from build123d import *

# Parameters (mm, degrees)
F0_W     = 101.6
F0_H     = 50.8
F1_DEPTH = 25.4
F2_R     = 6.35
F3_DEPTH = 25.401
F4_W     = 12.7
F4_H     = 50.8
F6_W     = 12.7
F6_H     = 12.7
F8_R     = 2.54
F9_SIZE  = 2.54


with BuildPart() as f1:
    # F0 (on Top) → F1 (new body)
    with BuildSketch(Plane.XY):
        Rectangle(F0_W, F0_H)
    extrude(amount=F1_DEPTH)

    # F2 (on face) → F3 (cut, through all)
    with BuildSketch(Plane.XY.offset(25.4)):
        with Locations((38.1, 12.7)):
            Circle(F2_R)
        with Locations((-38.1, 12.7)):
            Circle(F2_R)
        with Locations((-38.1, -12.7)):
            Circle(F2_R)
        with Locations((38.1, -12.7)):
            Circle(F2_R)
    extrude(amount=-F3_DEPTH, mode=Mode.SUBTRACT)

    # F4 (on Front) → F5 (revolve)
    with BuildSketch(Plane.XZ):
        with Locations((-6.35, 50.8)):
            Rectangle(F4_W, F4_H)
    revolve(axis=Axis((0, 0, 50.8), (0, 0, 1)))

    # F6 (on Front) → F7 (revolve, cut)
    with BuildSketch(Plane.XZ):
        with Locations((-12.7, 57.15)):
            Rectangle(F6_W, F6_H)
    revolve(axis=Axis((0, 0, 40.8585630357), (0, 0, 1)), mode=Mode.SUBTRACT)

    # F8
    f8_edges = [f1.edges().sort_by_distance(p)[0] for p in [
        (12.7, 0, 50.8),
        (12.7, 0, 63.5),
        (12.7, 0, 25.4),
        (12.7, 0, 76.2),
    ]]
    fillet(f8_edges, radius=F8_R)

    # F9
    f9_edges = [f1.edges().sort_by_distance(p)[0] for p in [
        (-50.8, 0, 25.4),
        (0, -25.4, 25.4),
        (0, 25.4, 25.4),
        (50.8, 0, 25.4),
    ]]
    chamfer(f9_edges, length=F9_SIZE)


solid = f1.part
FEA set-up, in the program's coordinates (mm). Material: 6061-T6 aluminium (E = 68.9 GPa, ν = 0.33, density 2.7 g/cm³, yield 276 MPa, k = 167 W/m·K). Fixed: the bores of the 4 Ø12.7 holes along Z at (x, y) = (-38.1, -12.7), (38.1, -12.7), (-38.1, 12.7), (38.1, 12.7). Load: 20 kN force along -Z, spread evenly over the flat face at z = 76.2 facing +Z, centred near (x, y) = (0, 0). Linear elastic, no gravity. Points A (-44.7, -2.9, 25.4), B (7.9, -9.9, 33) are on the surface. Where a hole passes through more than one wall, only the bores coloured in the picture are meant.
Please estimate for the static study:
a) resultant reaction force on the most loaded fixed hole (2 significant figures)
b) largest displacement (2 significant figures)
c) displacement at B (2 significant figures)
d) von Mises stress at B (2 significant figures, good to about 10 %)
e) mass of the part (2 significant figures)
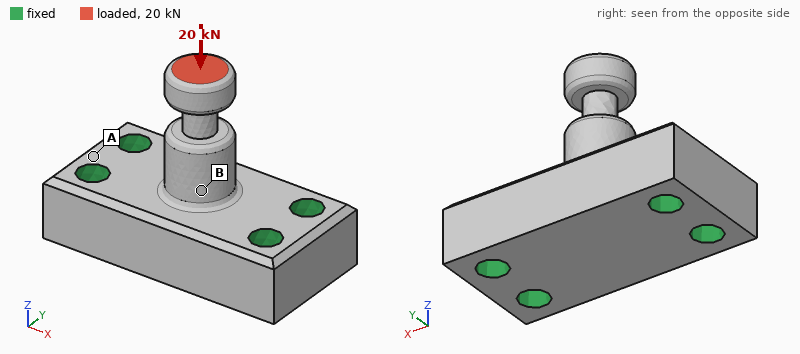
5.1 kN
81 µm
20 µm
37 MPa
370 g
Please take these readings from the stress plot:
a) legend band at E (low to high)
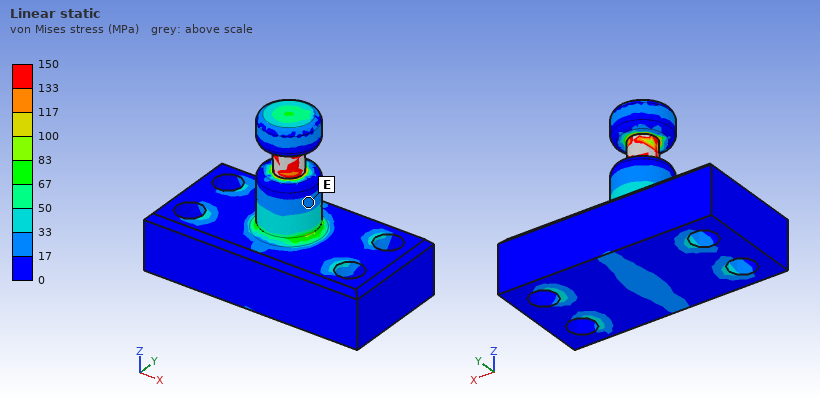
17 to 33 MPa
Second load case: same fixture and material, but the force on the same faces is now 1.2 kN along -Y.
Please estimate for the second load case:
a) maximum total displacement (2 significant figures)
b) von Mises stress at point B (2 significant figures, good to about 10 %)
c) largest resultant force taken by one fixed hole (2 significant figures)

0.16 mm
24 MPa
1000 N
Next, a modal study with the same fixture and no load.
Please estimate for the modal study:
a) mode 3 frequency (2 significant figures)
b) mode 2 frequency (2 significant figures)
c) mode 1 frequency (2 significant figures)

8400 Hz
4200 Hz
4100 Hz
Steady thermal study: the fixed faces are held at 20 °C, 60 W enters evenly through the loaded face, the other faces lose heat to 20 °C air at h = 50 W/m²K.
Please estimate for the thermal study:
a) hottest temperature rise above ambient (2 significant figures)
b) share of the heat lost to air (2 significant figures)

75 K
14 %
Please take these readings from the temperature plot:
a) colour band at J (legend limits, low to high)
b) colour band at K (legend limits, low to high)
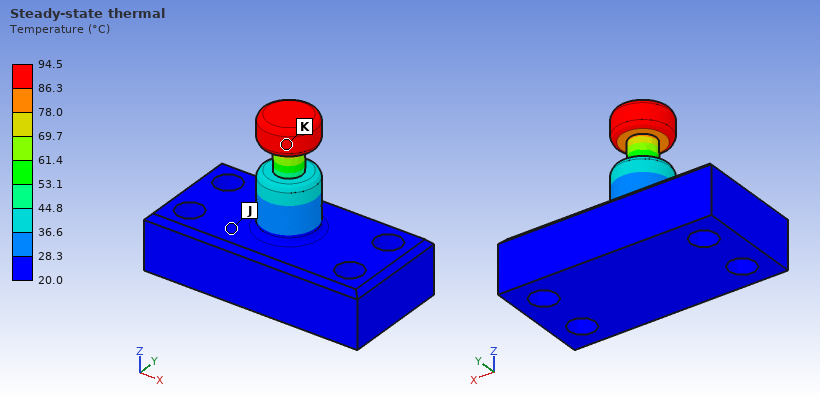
20.0 to 28.3 °C
86.3 to 94.5 °C
